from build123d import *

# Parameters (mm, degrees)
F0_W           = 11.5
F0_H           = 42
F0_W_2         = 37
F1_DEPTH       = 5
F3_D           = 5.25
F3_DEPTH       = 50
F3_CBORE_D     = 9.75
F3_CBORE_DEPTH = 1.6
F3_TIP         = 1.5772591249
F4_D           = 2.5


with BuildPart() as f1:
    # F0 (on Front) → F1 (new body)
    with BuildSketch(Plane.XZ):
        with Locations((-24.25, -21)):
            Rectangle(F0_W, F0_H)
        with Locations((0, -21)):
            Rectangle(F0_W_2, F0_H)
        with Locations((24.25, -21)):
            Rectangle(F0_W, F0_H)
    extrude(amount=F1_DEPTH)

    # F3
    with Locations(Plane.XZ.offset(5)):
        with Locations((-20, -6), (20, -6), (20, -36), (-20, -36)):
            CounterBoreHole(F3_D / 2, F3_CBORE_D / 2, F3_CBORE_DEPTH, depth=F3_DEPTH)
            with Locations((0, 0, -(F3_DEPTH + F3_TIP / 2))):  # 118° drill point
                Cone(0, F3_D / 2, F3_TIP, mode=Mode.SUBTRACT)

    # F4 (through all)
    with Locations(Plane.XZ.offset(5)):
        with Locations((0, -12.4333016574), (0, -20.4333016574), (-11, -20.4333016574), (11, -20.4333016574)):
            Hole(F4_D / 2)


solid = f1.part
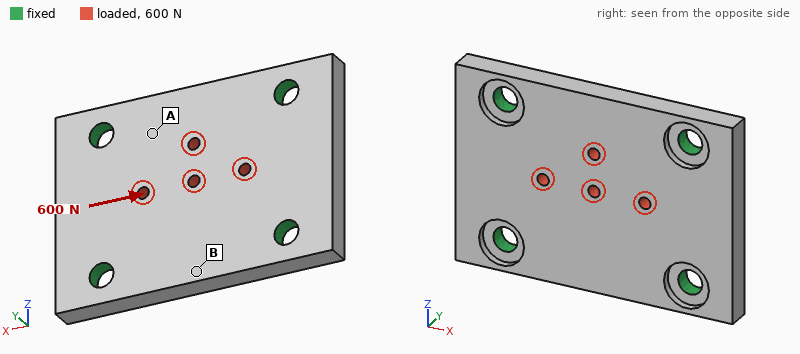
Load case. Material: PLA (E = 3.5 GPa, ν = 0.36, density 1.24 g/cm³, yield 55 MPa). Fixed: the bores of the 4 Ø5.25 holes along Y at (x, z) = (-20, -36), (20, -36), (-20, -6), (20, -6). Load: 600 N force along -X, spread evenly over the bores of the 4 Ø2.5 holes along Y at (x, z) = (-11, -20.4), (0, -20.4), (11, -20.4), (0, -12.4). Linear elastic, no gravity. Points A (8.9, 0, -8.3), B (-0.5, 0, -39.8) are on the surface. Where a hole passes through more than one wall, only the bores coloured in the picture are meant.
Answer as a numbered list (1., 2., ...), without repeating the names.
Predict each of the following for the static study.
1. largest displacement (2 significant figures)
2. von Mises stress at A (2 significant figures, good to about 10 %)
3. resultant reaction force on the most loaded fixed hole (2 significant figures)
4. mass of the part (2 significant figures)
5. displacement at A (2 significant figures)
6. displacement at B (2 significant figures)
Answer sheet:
1. 19 µm
2. 2.6 MPa
3. 170 N
4. 15 g
5. 8.0 µm
6. 4.2 µm
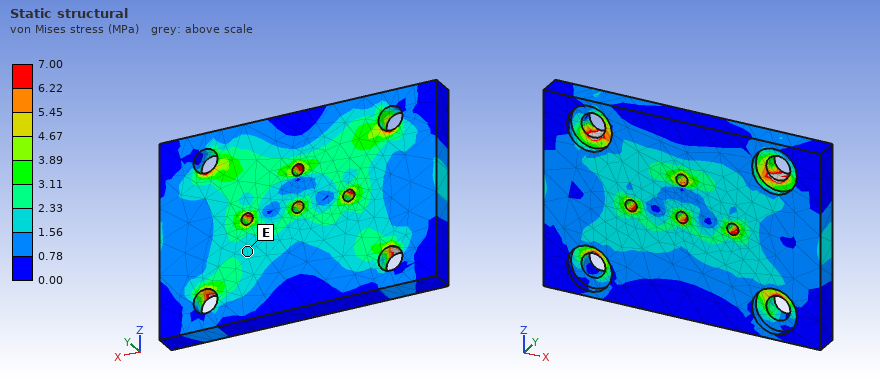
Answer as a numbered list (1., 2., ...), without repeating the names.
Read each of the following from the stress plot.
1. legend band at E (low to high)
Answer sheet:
1. 1.56 to 2.33 MPa
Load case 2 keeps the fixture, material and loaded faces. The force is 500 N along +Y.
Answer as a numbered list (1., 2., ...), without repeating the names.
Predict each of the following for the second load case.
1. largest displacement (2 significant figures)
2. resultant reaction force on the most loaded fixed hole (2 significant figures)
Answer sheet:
1. 0.20 mm
2. 180 N
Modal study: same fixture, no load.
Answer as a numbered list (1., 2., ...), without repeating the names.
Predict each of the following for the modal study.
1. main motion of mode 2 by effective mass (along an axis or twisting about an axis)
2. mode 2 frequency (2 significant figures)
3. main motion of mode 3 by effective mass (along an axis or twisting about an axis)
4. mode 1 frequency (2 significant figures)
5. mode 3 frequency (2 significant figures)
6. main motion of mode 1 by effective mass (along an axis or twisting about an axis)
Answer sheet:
1. twisting about X
2. 5500 Hz
3. along Y
4. 4100 Hz
5. 6700 Hz
6. along Y
